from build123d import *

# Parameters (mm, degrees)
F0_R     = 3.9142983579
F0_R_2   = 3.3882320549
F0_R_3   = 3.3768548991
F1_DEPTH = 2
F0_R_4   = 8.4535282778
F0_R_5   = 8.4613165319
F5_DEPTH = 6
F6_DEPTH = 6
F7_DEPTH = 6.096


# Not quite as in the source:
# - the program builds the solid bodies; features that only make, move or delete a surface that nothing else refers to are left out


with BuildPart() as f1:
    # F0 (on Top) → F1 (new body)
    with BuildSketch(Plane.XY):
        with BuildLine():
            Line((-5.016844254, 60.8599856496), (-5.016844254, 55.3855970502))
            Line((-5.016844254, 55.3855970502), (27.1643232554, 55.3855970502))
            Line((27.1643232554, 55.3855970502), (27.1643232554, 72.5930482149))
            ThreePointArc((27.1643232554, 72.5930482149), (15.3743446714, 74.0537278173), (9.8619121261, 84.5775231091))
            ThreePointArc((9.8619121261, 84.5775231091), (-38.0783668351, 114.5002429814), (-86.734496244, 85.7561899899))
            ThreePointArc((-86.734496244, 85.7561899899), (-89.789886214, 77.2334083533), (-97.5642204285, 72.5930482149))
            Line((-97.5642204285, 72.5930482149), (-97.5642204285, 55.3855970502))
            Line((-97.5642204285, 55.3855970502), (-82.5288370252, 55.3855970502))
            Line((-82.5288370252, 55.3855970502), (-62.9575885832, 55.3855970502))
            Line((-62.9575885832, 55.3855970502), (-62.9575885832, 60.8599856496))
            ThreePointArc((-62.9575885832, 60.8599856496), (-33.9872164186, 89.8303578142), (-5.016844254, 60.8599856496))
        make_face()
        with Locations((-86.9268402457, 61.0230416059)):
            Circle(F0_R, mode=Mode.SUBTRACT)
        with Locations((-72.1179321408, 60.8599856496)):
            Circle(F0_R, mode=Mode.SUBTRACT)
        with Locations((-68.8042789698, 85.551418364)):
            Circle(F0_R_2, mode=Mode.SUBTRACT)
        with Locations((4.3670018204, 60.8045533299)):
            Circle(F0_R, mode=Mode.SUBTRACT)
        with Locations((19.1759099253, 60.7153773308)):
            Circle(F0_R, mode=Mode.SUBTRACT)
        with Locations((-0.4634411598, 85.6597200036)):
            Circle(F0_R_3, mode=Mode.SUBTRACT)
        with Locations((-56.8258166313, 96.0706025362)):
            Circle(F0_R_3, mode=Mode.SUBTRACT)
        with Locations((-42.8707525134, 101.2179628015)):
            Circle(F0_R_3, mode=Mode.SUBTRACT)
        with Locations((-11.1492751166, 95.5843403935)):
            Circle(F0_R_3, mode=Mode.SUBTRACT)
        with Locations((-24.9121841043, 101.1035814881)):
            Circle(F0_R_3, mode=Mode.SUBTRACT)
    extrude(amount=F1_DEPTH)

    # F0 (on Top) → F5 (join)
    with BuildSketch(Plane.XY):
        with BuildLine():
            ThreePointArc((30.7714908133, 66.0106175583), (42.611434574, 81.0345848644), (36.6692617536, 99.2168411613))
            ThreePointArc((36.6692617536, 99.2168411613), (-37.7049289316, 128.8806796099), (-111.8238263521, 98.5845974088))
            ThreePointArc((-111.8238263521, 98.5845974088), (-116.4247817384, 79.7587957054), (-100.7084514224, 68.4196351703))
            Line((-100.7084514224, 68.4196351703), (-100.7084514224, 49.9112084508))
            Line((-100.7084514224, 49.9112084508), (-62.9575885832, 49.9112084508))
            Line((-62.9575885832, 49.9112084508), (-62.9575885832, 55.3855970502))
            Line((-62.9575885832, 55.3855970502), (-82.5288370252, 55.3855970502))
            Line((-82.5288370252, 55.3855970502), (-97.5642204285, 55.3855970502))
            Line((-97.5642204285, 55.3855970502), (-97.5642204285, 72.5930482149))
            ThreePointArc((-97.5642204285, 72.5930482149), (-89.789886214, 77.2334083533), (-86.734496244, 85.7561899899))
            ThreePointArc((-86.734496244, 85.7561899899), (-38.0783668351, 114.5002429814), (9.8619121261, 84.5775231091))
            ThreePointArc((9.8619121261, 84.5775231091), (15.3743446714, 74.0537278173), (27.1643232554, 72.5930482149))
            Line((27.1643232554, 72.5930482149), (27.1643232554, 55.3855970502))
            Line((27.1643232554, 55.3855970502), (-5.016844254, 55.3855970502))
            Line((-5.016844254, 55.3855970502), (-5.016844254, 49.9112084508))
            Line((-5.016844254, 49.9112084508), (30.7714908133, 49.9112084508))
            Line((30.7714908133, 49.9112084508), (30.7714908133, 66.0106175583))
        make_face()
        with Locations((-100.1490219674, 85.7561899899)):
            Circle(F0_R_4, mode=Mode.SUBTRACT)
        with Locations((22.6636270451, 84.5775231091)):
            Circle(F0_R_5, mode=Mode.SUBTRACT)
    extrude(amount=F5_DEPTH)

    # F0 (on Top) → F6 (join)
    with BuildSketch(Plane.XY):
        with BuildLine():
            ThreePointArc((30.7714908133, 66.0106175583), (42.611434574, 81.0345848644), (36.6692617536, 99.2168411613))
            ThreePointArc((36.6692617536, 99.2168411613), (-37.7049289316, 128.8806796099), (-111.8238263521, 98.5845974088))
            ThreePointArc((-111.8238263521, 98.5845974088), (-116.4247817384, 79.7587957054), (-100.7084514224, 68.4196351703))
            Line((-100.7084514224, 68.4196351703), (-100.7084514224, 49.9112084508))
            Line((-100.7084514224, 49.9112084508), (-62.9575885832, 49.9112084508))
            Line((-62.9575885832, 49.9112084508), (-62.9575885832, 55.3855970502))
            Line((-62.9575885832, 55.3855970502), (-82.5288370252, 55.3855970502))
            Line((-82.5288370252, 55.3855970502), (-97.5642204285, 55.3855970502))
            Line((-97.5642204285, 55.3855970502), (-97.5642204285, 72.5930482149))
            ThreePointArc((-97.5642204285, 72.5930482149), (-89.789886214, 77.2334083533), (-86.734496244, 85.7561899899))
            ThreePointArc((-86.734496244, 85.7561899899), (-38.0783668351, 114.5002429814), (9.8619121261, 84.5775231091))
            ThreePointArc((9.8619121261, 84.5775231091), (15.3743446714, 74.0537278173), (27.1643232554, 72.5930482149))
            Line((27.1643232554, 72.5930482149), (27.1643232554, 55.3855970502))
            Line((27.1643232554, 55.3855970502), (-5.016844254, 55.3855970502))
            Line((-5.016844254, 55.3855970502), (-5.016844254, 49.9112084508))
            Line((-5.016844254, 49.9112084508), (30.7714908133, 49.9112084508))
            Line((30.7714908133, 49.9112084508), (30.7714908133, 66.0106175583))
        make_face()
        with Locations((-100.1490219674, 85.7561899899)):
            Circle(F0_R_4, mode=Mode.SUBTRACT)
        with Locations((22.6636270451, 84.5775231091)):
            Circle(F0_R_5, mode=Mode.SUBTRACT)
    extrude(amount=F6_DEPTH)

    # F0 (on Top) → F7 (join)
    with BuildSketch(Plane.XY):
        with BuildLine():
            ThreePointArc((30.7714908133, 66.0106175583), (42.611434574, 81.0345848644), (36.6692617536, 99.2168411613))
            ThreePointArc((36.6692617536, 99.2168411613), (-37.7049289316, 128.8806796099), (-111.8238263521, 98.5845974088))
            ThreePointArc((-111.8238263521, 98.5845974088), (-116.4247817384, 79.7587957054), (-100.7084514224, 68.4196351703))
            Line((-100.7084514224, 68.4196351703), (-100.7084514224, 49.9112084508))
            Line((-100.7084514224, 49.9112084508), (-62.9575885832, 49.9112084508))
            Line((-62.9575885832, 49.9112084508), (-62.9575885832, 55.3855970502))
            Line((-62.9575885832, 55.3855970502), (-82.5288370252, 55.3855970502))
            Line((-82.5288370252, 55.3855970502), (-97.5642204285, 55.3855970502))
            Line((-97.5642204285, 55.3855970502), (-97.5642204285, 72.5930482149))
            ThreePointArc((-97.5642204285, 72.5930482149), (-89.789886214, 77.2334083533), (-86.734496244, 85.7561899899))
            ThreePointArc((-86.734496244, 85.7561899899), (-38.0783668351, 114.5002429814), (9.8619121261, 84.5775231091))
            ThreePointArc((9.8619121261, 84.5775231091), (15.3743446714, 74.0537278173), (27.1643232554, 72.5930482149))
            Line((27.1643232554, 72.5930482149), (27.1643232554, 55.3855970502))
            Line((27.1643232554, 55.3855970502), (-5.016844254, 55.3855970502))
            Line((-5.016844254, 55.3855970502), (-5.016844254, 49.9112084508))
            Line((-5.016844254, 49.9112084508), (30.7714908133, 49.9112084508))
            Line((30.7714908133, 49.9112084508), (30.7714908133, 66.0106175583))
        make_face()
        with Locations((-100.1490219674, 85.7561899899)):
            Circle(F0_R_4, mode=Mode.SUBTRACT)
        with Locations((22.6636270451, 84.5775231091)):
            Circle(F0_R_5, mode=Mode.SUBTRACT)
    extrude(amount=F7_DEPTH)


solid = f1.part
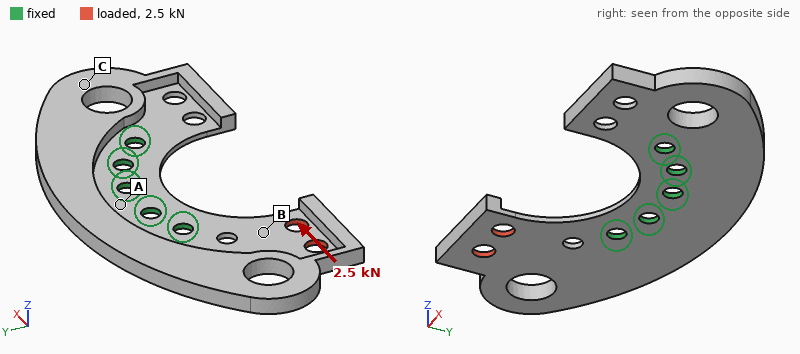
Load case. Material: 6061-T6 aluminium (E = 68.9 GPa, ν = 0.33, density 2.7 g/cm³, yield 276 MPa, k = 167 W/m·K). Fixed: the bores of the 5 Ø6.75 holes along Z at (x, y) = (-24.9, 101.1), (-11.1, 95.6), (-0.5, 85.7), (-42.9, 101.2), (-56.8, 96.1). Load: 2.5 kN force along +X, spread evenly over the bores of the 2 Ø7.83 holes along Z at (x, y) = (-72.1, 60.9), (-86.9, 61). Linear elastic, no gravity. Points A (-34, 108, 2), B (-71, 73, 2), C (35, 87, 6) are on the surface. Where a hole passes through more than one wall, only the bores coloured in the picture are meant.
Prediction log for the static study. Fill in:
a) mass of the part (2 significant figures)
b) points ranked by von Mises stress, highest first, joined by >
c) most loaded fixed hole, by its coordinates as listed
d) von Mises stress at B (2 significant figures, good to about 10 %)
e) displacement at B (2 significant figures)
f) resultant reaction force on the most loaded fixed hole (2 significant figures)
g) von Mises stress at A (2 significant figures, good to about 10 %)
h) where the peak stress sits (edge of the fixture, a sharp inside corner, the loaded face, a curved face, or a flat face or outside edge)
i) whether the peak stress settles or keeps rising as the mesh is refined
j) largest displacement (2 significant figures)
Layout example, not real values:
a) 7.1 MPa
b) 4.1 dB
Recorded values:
a) 85 g
b) B > A > C
c) (-56.8, 96.1)
d) 95 MPa
e) 0.16 mm
f) 4.0 kN
g) 40 MPa
h) edge of the fixture
i) keeps rising
j) 0.49 mm
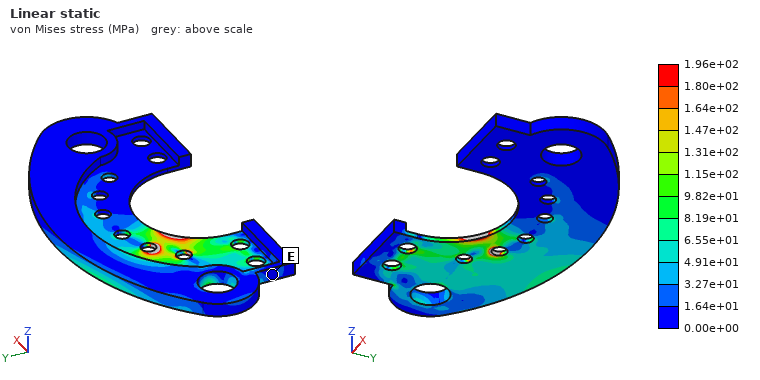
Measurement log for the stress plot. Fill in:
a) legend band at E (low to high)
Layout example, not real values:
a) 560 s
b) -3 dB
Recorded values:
a) 0.00e+00 to 1.64e+01 MPa
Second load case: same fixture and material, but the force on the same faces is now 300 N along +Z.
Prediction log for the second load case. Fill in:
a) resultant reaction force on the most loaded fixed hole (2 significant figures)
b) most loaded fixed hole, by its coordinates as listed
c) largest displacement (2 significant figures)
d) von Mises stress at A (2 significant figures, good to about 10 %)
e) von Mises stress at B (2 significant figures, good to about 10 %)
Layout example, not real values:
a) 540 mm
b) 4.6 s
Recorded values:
a) 610 N
b) (-56.8, 96.1)
c) 1.6 mm
d) 50 MPa
e) 77 MPa
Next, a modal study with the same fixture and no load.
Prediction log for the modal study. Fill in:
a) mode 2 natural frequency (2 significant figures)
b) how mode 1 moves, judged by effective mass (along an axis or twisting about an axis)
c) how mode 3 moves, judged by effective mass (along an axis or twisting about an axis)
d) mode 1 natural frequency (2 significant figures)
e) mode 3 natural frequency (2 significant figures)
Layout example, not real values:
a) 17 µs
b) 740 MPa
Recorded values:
a) 1000 Hz
b) along Z
c) along Z
d) 680 Hz
e) 1400 Hz
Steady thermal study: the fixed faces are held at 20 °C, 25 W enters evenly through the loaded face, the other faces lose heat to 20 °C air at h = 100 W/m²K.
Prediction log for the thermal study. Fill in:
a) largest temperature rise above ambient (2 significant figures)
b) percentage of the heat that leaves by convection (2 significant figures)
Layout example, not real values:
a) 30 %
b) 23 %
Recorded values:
a) 47 K
b) 62 %
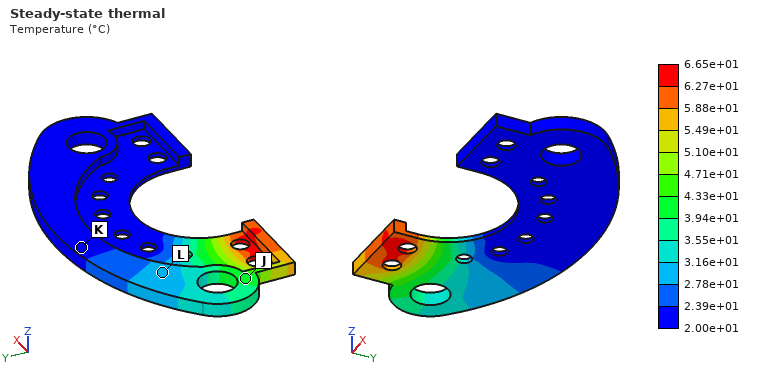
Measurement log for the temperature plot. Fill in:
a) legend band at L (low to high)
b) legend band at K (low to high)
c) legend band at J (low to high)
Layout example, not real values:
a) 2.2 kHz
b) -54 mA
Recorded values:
a) 2.78e+01 to 3.16e+01 °C
b) 2.00e+01 to 2.39e+01 °C
c) 3.94e+01 to 4.33e+01 °C
